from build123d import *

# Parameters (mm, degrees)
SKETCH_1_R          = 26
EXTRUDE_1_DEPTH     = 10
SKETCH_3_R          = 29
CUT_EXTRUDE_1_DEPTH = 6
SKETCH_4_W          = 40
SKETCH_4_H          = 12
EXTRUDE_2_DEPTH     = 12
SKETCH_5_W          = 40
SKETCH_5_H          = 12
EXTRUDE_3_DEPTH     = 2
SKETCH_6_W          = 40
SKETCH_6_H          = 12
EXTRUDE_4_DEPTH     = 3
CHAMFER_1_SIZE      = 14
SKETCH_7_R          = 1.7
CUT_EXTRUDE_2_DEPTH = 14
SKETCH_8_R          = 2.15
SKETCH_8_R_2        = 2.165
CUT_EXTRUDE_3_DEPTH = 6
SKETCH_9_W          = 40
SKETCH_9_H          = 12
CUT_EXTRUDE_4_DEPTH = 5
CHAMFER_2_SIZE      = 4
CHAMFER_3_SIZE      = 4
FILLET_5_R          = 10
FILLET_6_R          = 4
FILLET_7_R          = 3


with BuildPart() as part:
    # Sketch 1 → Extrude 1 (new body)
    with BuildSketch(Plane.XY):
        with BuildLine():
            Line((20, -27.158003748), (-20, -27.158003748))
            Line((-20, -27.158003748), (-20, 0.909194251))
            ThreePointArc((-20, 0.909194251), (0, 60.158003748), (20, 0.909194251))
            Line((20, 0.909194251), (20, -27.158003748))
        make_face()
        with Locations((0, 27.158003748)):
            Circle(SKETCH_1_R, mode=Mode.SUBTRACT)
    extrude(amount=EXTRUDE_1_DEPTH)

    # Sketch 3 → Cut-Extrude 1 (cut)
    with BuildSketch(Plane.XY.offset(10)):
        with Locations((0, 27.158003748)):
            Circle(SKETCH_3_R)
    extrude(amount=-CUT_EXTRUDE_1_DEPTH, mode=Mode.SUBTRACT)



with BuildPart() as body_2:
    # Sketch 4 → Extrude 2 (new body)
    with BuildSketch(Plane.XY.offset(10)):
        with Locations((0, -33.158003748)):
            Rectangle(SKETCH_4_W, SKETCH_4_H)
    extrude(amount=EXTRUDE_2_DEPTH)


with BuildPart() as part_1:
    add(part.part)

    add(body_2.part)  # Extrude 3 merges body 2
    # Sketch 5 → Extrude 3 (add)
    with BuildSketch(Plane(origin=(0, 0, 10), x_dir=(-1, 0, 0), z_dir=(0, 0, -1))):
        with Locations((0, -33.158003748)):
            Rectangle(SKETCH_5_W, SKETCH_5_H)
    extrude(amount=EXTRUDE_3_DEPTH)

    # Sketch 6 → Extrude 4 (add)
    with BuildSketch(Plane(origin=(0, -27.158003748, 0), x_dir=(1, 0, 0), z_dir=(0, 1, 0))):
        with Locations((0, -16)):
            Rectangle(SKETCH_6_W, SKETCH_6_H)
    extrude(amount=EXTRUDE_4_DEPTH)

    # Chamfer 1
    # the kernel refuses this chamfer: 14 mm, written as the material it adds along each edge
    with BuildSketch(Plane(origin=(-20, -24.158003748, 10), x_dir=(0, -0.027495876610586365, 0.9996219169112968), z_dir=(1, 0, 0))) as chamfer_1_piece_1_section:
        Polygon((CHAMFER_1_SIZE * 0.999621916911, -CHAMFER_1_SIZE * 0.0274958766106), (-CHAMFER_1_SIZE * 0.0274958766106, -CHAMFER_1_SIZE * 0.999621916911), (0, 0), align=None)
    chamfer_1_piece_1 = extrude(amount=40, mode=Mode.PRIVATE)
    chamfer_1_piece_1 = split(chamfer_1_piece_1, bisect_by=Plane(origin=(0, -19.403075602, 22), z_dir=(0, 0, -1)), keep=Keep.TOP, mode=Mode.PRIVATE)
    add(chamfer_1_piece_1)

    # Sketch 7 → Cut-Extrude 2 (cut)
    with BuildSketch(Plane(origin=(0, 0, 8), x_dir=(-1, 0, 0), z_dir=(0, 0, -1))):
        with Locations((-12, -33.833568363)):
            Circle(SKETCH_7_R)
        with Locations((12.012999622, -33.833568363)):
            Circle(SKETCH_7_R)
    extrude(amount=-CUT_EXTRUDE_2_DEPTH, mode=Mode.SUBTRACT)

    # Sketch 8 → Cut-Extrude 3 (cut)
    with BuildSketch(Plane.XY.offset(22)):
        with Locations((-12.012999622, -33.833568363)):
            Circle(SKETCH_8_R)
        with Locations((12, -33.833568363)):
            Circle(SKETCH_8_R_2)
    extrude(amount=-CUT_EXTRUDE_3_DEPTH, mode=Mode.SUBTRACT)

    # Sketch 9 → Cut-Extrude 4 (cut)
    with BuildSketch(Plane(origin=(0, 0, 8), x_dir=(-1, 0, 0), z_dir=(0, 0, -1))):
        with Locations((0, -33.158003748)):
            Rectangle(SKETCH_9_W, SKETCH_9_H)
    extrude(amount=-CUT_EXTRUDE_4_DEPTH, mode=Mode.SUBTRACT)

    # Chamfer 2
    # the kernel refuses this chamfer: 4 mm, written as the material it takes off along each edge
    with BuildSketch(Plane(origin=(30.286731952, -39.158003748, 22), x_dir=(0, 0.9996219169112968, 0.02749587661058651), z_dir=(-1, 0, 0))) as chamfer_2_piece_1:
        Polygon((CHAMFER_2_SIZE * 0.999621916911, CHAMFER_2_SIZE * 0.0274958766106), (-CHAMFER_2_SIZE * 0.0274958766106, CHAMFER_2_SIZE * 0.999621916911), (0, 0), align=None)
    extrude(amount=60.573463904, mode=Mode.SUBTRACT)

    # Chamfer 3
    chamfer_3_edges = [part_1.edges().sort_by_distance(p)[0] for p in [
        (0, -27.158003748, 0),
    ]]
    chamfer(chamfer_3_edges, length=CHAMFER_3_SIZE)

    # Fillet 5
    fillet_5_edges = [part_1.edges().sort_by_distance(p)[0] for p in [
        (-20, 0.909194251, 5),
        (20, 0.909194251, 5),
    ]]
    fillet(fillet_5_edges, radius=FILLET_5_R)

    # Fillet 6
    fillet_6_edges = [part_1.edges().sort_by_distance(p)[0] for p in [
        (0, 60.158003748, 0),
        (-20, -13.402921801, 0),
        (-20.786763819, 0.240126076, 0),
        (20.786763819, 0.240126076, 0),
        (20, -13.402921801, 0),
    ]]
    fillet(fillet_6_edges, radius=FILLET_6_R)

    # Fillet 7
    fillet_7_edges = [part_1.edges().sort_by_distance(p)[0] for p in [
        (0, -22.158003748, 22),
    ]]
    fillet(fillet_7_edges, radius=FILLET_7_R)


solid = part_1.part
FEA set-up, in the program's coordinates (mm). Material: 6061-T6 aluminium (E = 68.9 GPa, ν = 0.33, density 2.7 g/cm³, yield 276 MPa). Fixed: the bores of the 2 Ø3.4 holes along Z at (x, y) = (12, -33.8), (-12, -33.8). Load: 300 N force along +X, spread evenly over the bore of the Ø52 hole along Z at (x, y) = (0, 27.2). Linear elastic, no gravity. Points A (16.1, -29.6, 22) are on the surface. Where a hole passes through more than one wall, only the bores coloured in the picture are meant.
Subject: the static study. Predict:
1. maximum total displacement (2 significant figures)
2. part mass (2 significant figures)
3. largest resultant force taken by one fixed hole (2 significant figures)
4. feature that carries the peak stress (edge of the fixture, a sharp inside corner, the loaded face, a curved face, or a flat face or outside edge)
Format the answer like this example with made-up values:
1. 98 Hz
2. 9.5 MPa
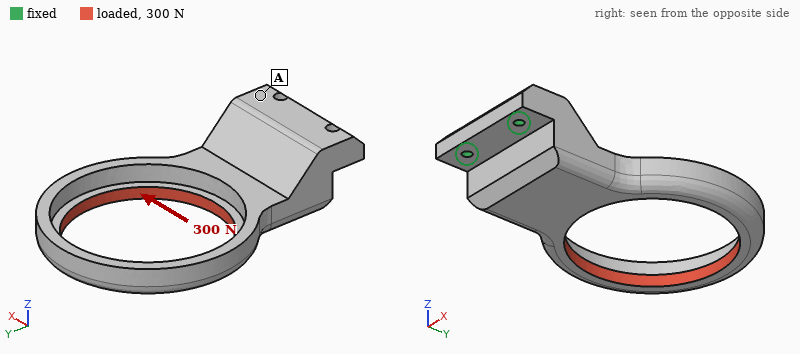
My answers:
1. 0.20 mm
2. 74 g
3. 750 N
4. edge of the fixture
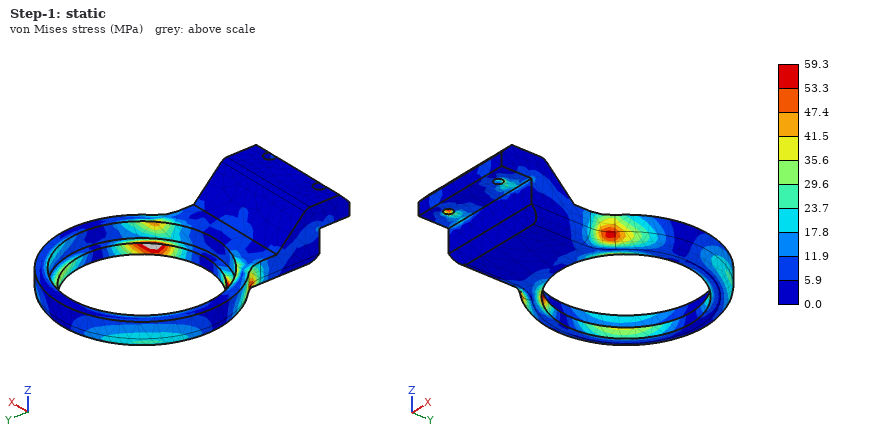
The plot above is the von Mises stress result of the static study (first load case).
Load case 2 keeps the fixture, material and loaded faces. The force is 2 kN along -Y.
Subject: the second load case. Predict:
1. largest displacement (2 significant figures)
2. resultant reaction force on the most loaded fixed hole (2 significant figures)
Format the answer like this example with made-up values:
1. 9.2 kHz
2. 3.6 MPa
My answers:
1. 0.90 mm
2. 1.0 kN
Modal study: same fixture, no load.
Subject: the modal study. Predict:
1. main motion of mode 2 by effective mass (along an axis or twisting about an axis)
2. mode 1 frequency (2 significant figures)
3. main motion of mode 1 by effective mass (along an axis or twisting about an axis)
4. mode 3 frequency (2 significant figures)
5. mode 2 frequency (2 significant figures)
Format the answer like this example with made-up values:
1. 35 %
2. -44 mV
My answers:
1. along X
2. 700 Hz
3. along Z
4. 2400 Hz
5. 1300 Hz
